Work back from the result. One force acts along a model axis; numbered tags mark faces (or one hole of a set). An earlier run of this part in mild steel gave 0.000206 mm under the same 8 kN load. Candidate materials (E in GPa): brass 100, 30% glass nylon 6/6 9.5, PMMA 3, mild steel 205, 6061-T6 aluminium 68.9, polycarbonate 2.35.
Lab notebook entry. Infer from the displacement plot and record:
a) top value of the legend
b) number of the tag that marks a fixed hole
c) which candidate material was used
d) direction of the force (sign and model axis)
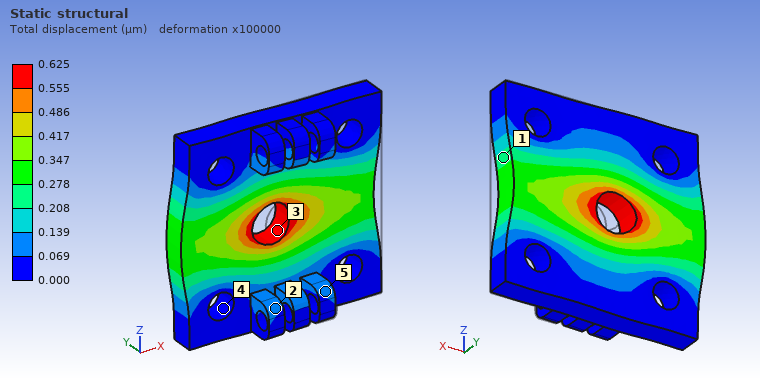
0.625 µm
4
6061-T6 aluminium
-X
